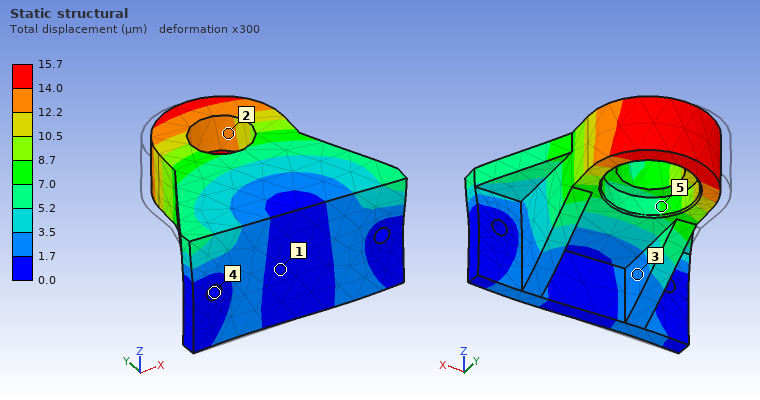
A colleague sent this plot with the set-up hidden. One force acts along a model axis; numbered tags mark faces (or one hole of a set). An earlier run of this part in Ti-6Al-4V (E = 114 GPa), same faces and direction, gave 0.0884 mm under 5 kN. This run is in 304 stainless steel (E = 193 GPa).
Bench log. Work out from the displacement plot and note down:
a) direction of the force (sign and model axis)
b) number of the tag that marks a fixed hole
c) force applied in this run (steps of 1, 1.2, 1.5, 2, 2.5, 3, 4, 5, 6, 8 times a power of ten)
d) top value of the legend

+X
4
1.5 kN
15.7 µm
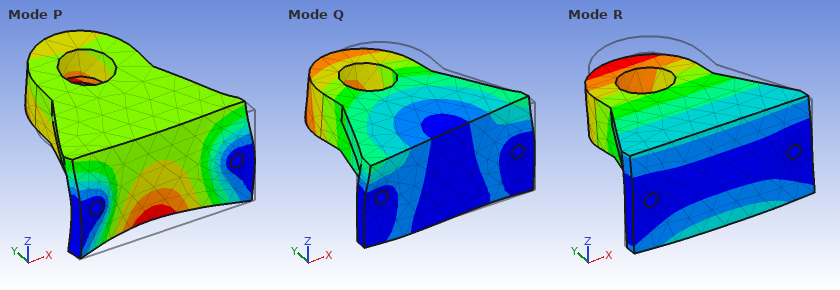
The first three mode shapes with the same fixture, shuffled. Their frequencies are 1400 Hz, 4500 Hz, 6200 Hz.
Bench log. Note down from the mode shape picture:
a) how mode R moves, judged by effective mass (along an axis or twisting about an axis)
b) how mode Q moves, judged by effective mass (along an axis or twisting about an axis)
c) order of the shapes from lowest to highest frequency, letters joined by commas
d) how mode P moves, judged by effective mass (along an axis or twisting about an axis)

along Z
along X
R, Q, P
along Y
